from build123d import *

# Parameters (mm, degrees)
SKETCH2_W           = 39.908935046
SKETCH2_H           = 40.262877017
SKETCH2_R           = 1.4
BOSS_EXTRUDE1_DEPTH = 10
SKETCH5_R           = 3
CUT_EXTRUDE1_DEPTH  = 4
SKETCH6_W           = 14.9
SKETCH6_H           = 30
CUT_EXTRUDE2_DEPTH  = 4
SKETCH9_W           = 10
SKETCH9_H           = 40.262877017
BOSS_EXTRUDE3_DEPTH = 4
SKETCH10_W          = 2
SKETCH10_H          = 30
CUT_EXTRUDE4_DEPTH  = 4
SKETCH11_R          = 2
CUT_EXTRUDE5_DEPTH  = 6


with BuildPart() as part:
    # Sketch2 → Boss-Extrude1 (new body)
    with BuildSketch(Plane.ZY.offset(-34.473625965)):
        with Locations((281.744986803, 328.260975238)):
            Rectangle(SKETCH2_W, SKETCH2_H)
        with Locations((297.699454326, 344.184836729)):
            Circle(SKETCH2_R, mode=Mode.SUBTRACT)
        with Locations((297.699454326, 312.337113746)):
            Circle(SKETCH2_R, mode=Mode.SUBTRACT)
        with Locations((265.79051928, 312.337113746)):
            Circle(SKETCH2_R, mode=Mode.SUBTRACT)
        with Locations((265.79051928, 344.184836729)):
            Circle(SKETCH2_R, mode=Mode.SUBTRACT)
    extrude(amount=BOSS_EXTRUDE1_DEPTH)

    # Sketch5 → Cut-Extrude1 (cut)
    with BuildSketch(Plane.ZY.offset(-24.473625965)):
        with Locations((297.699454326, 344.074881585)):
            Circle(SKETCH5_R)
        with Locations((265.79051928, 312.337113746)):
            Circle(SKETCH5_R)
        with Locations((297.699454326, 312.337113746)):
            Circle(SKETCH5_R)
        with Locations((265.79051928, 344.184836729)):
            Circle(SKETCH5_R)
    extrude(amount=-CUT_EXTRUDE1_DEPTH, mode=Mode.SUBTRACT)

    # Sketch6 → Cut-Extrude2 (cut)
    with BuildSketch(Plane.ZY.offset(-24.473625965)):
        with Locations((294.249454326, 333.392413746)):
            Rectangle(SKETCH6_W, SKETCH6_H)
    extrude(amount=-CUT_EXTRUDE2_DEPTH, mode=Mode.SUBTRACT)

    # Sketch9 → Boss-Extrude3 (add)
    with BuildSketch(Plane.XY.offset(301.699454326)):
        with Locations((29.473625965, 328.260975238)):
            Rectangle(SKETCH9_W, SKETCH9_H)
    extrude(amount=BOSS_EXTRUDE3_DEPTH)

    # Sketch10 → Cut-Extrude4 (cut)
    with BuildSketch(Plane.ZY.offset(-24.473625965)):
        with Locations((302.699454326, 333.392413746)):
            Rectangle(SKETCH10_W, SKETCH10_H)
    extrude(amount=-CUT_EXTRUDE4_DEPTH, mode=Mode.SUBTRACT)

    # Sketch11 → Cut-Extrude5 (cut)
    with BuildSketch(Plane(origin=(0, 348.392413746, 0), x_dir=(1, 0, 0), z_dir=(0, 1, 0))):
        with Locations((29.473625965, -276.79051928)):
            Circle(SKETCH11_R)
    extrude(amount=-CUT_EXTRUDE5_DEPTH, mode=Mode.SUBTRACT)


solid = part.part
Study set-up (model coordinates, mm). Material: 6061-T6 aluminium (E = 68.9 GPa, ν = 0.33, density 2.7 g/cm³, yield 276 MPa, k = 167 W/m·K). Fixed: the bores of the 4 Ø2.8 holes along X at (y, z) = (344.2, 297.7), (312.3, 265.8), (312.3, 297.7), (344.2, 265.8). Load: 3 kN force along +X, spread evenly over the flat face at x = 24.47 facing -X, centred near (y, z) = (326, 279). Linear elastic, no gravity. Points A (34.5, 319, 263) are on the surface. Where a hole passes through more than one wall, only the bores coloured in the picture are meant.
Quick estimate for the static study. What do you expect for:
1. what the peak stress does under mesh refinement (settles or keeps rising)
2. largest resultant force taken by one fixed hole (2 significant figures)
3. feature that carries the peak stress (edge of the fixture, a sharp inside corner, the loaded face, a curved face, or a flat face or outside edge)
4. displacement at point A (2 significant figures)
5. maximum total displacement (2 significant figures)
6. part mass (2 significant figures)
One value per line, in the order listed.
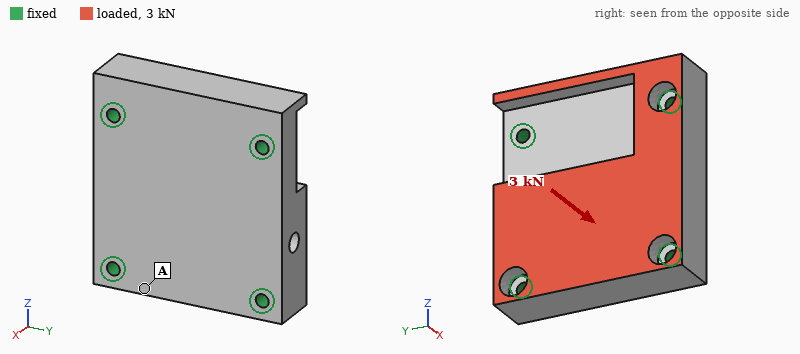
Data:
keeps rising
930 N
edge of the fixture
3.0 µm
7.3 µm
41 g
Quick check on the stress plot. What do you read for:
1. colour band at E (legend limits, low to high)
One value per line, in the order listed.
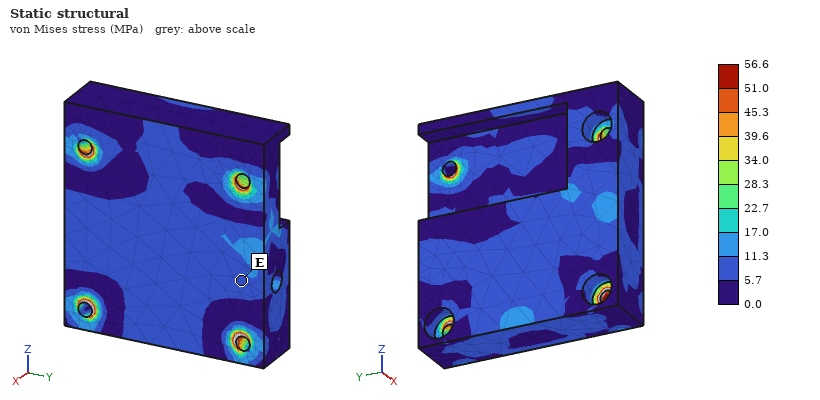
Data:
5.7 to 11.3 MPa
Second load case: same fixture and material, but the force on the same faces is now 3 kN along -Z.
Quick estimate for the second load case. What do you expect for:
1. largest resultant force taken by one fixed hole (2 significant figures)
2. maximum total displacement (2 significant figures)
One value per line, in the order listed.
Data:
970 N
8.0 µm
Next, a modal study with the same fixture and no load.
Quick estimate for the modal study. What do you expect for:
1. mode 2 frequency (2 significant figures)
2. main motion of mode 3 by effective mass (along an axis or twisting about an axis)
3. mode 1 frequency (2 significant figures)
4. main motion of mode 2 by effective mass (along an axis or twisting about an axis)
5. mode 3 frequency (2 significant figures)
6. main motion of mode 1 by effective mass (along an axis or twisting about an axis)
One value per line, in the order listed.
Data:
25 kHz
twisting about Z
19 kHz
twisting about Y
28 kHz
along X
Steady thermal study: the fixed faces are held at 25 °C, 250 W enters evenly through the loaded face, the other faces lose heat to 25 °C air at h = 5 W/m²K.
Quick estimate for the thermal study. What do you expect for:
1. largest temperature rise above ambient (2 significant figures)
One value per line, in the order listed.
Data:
40 K
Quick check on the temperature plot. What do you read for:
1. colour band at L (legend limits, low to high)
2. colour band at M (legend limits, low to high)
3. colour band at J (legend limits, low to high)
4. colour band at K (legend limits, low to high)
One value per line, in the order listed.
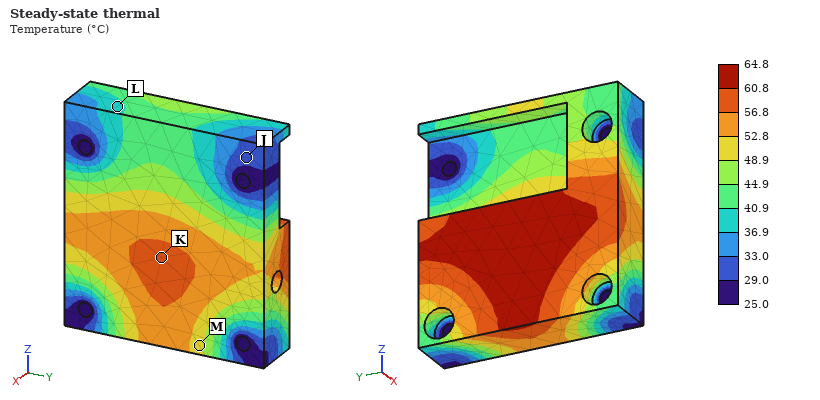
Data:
36.9 to 40.9 °C
48.9 to 52.8 °C
29.0 to 33.0 °C
56.8 to 60.8 °C
